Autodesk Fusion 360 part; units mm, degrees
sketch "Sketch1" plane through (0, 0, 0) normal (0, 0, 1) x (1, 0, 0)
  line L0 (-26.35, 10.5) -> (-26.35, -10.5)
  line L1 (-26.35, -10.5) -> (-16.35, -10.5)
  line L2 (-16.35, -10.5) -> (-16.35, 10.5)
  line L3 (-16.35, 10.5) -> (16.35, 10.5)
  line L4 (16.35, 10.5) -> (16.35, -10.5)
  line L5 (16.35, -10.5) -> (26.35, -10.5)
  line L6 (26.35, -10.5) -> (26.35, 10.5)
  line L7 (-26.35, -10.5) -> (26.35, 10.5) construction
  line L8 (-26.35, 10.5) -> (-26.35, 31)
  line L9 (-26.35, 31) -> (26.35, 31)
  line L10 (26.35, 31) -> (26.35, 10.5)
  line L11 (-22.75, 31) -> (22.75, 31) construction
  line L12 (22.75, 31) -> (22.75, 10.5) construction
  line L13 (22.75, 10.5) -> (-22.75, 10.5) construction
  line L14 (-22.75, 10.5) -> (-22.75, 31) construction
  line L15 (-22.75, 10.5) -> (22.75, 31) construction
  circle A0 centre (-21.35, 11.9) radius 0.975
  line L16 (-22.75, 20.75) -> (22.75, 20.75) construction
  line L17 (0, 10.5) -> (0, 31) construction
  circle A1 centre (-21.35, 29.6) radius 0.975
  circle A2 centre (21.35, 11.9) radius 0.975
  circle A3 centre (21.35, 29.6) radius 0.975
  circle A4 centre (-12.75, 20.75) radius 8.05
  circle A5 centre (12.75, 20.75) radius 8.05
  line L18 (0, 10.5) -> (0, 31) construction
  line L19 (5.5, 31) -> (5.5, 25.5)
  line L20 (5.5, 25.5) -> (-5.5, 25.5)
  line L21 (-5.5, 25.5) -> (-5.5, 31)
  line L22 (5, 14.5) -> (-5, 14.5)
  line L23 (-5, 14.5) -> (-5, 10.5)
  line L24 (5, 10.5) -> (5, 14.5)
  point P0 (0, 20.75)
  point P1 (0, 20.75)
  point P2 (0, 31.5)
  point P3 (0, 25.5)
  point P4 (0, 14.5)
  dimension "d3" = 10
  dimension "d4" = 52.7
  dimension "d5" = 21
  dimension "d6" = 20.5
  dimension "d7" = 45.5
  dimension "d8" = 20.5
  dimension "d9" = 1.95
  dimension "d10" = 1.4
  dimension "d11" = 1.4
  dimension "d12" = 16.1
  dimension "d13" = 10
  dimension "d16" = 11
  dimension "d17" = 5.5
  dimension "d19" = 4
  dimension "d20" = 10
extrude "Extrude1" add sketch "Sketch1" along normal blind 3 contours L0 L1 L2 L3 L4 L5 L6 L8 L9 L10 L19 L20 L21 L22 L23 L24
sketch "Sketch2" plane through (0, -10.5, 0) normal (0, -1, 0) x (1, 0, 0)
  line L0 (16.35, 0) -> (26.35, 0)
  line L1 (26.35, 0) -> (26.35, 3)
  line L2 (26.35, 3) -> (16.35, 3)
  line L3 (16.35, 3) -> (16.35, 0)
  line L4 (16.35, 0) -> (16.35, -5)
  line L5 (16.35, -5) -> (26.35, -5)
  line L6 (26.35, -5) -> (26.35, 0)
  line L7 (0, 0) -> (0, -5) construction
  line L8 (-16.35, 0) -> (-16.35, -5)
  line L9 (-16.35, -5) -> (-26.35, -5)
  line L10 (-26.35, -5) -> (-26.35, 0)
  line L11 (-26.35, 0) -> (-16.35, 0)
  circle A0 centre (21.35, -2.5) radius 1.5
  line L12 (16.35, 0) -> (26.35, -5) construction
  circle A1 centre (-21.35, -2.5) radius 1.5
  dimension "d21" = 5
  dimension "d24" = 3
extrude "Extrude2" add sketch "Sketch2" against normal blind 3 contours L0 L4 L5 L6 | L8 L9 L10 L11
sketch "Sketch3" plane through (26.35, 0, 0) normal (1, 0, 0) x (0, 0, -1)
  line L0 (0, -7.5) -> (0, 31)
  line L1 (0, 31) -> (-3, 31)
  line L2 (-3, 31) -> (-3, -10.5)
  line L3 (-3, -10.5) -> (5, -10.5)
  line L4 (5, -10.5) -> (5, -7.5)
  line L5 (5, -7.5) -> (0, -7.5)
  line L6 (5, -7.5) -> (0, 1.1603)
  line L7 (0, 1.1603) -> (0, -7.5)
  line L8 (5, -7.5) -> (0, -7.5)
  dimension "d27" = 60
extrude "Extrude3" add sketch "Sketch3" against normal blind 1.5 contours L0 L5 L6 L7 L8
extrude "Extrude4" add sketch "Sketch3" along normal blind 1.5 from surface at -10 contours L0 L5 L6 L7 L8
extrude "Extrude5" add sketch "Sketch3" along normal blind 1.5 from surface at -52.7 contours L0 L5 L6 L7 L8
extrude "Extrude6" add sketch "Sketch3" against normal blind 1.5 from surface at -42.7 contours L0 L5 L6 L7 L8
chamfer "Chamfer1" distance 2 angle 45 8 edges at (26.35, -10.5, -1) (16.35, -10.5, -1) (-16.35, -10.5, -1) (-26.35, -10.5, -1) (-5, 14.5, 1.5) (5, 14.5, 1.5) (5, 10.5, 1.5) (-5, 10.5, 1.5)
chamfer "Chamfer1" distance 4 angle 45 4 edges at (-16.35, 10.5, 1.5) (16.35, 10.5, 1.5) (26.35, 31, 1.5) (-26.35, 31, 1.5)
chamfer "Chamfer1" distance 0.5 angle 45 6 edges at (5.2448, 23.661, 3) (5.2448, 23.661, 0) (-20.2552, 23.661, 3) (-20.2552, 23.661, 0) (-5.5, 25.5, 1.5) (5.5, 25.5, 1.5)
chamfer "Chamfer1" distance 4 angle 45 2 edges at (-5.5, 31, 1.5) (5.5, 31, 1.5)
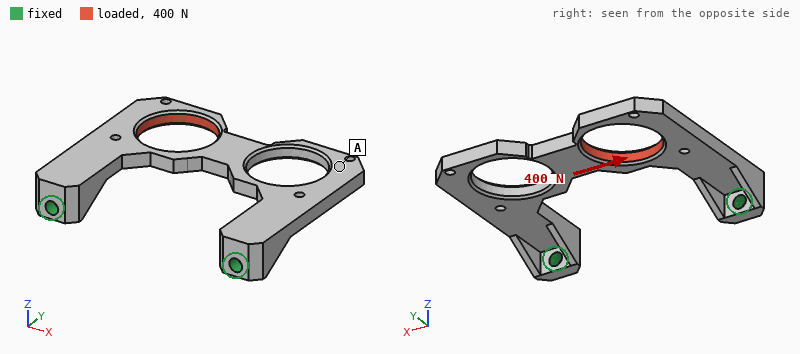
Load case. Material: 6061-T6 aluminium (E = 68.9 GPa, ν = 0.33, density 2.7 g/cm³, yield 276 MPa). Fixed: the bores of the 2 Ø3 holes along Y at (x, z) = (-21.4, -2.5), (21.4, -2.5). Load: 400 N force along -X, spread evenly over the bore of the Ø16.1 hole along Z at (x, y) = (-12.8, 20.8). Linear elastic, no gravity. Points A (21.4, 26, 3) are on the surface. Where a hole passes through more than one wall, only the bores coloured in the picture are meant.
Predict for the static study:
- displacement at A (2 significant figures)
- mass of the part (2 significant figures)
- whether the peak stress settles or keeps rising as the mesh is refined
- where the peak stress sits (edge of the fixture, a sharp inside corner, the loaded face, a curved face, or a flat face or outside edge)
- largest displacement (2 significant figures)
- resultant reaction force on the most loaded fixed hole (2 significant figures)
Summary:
0.070 mm
8.6 g
keeps rising
edge of the fixture
0.10 mm
270 N
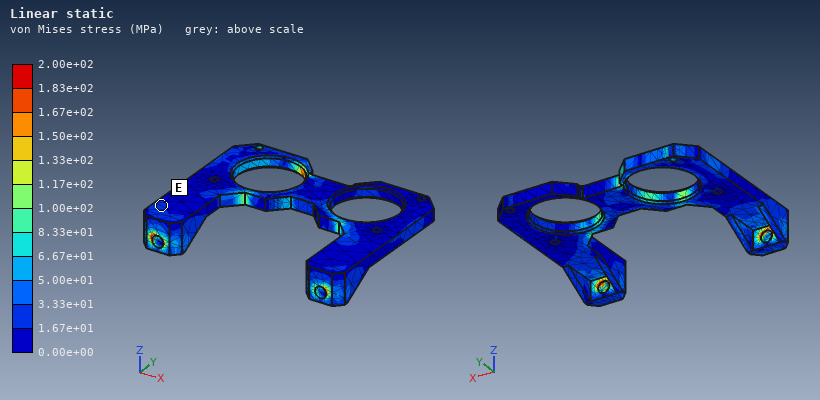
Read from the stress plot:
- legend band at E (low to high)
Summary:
1.67e+01 to 3.33e+01 MPa
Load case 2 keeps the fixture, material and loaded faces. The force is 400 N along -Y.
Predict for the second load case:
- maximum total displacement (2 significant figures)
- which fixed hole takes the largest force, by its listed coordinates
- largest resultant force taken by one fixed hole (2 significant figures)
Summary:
47 µm
(-21.4, -2.5)
330 N
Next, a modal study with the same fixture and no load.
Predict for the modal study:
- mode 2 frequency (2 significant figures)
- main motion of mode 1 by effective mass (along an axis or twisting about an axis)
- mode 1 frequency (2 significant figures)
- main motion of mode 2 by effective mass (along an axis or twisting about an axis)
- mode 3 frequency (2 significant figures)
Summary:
2700 Hz
along Z
1600 Hz
twisting about Y
5200 Hz
